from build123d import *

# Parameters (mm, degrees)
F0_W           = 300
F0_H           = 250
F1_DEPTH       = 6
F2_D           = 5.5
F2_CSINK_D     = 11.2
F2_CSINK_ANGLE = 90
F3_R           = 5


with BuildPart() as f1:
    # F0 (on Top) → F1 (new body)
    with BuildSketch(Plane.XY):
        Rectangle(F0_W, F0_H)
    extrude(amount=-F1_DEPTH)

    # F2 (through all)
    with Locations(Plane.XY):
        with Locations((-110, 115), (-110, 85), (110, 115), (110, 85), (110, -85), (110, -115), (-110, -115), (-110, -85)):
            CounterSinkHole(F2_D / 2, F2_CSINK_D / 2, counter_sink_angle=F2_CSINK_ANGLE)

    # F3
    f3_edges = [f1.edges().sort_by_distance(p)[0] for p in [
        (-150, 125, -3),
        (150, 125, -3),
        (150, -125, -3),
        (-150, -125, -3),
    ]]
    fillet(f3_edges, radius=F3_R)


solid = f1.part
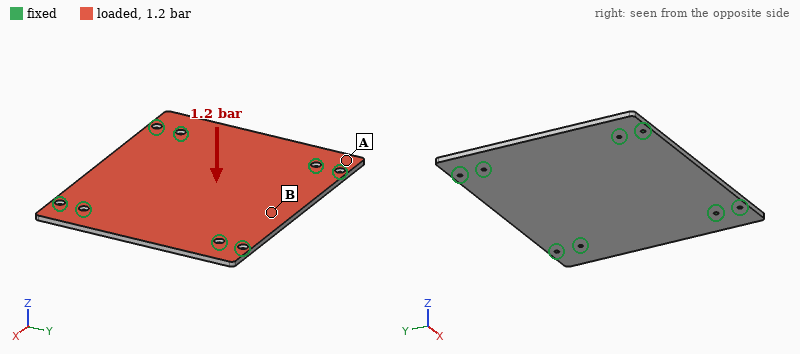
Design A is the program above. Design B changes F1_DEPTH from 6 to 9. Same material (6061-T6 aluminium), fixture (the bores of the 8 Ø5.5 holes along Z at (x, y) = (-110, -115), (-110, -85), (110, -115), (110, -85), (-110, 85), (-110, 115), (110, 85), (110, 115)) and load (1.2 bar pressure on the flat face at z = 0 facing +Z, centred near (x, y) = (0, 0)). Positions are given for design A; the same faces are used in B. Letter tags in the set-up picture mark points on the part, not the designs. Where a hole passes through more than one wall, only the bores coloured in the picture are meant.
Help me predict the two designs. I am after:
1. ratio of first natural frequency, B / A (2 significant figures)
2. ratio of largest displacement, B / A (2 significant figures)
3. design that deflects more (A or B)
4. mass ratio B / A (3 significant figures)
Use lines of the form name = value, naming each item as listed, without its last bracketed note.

ratio of first natural frequency, B / A = 1.5
ratio of largest displacement, B / A = 0.30
design that deflects more = A
mass ratio B / A = 1.50
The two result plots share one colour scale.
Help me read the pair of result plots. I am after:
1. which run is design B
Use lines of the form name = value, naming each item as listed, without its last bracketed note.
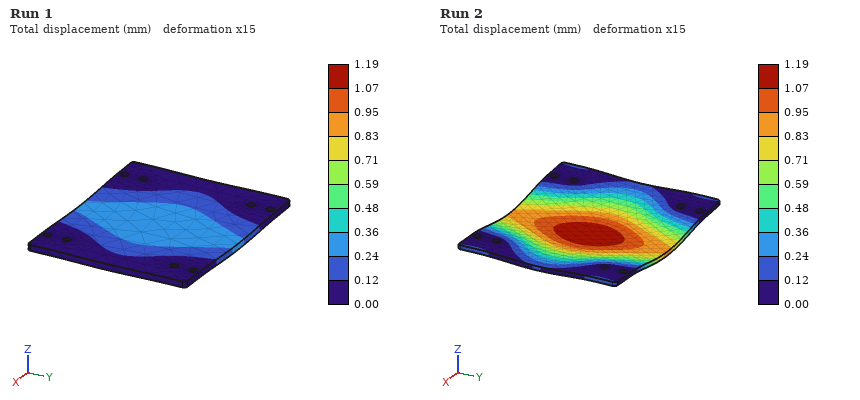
which run is design B = Run 1
